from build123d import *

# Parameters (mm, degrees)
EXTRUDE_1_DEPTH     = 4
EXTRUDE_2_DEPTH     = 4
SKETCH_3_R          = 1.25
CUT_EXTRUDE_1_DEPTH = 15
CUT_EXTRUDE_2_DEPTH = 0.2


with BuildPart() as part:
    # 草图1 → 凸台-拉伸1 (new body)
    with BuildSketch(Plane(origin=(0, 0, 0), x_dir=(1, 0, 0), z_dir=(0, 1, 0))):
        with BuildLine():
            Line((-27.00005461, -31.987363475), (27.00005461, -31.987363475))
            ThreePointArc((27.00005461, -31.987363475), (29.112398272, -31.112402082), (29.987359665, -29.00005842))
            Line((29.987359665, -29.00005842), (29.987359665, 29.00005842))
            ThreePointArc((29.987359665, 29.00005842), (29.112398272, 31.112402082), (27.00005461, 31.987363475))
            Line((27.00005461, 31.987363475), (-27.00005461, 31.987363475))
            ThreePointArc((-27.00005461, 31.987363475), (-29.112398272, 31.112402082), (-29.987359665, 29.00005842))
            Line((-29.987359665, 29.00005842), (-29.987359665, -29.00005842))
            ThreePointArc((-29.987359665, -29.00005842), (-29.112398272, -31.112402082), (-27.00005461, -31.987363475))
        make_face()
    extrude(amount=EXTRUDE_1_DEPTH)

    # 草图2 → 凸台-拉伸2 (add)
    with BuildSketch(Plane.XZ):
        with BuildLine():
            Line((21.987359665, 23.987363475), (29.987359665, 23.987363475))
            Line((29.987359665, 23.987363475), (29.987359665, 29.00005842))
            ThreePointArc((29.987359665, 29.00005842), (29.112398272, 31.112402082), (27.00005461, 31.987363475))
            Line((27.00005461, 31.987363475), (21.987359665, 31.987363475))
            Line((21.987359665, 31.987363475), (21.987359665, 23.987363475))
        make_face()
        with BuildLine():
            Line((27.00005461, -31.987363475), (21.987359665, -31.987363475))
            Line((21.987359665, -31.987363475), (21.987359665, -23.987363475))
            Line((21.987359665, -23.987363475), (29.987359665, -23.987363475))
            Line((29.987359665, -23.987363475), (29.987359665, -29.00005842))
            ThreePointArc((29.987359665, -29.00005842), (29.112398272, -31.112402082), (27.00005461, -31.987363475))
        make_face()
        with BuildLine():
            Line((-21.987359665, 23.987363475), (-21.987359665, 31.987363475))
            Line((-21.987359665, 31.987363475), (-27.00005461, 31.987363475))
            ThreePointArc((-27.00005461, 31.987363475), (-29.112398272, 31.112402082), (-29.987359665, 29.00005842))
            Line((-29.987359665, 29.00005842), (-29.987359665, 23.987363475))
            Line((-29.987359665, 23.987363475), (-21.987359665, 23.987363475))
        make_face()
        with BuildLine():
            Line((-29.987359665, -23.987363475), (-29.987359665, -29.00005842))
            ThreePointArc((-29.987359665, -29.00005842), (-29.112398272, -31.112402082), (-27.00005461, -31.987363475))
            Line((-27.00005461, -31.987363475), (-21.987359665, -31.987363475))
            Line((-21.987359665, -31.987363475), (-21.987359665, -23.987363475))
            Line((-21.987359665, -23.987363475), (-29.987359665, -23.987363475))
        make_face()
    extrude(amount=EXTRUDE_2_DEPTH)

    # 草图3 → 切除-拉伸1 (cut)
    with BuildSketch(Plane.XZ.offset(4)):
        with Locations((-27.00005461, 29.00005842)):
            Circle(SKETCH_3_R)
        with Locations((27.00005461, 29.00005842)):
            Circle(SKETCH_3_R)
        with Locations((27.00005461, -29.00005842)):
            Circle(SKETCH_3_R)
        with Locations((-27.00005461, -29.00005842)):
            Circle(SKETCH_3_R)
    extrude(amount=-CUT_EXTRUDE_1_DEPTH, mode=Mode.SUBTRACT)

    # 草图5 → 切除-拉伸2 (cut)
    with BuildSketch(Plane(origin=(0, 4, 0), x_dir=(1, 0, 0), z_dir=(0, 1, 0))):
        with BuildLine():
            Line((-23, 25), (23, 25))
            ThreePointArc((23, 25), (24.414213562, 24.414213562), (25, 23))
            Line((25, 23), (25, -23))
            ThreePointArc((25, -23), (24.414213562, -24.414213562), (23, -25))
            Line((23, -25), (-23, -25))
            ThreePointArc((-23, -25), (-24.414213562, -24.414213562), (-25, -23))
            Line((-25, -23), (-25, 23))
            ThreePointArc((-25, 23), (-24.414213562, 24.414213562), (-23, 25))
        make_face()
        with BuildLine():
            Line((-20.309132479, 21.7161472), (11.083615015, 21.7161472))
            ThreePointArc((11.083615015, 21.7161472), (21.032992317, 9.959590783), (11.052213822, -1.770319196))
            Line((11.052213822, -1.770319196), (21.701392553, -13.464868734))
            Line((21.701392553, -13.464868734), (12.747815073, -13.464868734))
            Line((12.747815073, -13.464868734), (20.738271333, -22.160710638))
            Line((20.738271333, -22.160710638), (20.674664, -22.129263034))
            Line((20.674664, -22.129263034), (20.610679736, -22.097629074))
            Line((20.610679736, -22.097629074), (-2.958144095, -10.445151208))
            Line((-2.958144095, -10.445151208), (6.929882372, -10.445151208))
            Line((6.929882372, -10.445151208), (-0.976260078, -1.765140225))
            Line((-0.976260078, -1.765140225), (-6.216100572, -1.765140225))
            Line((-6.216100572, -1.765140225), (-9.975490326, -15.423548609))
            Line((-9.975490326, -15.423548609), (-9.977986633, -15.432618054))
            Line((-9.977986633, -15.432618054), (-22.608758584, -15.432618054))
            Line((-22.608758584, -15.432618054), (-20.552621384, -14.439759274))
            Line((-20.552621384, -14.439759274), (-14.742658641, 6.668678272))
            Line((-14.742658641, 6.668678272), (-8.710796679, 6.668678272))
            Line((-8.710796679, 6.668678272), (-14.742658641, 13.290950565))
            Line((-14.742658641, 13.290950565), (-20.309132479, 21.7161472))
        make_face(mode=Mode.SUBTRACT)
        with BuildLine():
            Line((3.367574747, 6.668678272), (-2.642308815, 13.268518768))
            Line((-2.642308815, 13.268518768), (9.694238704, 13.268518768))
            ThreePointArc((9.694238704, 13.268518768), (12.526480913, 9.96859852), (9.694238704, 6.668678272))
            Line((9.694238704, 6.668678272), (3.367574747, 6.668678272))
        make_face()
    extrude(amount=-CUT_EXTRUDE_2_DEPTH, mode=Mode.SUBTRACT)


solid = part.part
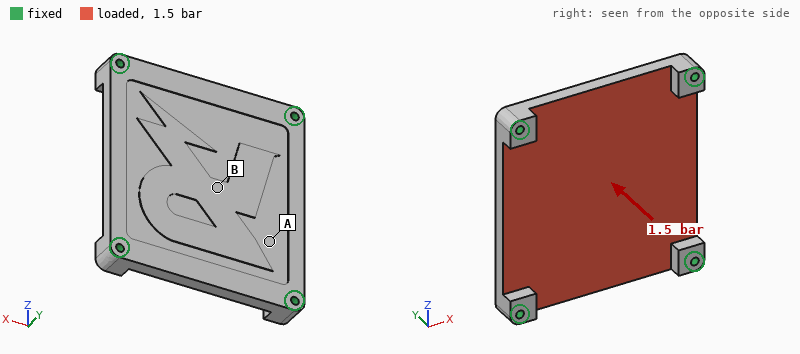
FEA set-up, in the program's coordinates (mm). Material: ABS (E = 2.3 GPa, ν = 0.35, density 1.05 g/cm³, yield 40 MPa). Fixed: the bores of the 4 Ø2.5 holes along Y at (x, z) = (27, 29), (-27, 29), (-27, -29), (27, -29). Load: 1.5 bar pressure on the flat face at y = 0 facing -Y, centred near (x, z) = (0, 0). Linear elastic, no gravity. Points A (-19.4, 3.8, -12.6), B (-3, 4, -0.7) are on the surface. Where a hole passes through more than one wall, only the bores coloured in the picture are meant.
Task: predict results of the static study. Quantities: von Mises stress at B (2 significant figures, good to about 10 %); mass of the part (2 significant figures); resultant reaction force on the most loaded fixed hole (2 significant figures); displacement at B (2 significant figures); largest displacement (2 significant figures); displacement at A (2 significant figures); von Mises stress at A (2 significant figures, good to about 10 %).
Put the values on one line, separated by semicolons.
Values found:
8.9 MPa; 17 g; 150 N; 0.70 mm; 0.70 mm; 0.39 mm; 5.2 MPa
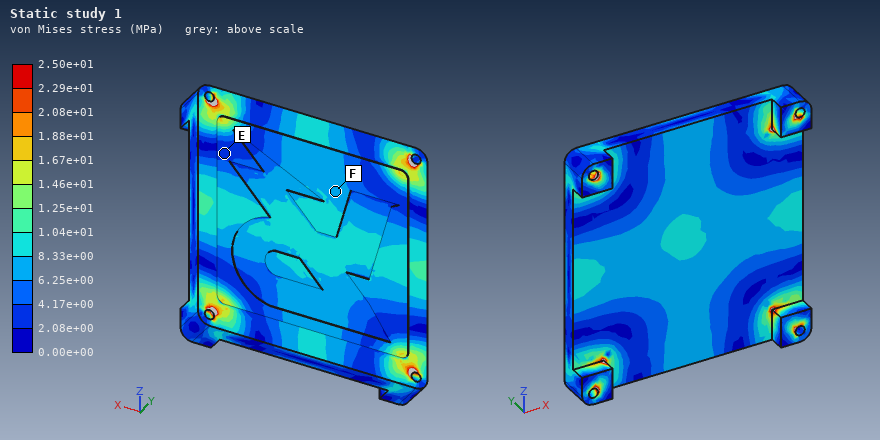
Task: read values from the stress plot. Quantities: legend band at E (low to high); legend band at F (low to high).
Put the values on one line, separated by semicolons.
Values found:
2.08e+00 to 4.17e+00 MPa; 6.25e+00 to 8.33e+00 MPa
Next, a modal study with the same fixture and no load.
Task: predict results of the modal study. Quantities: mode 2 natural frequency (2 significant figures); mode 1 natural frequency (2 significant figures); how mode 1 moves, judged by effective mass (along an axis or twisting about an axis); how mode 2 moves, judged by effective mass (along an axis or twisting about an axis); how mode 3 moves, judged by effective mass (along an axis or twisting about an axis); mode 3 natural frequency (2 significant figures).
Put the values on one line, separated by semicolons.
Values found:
2200 Hz; 1400 Hz; along Y; twisting about Z; twisting about X; 2500 Hz
